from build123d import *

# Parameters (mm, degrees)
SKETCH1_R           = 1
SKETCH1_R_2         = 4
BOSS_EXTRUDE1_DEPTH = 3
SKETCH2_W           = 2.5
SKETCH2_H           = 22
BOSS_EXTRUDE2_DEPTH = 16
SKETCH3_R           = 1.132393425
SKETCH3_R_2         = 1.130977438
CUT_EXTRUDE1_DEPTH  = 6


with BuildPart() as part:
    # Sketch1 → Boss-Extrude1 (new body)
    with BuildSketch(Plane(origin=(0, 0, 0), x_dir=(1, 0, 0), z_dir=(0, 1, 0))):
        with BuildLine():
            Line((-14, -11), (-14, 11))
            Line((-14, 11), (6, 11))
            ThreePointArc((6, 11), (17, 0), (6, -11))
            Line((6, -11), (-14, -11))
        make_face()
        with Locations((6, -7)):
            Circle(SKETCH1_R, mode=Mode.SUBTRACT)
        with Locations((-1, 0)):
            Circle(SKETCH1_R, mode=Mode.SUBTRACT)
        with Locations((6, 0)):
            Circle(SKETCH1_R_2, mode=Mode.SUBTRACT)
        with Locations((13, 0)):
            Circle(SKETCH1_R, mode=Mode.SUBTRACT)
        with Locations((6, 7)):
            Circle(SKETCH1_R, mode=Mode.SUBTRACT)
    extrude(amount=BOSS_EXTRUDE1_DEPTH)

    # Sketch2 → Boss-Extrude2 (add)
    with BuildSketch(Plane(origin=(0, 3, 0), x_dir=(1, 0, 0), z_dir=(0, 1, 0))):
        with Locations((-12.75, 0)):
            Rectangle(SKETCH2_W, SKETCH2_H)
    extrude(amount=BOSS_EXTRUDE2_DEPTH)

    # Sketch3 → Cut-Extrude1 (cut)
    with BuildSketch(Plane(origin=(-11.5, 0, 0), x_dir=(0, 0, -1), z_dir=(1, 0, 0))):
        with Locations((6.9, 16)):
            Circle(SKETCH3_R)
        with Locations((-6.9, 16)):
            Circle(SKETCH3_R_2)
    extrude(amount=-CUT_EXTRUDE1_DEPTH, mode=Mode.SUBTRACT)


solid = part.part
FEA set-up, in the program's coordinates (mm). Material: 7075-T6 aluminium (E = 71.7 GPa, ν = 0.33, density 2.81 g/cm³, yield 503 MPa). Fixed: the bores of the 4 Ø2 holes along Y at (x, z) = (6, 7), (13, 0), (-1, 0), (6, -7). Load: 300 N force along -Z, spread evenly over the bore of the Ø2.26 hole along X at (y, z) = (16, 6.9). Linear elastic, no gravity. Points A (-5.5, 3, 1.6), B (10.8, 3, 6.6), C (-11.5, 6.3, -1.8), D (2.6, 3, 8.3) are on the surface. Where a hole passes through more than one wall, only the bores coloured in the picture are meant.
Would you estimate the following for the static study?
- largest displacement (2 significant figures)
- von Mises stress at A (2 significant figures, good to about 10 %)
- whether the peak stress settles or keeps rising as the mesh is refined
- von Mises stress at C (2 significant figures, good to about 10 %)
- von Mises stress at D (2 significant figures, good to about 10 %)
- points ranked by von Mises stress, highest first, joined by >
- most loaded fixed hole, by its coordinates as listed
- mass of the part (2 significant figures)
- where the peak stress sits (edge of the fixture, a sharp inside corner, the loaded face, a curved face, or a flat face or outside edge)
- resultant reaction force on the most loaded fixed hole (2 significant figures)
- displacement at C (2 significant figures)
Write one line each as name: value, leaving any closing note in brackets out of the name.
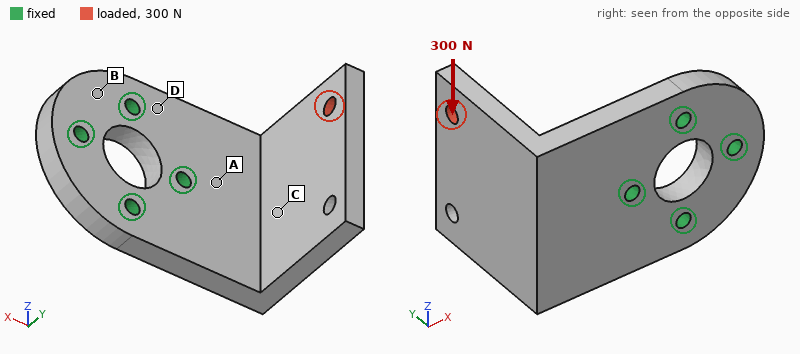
largest displacement: 0.20 mm
von Mises stress at A: 110 MPa
whether the peak stress settles or keeps rising as the mesh is refined: keeps rising
von Mises stress at C: 41 MPa
von Mises stress at D: 68 MPa
points ranked by von Mises stress, highest first, joined by >: A > D > C > B
most loaded fixed hole, by its coordinates as listed: (-1, 0)
mass of the part: 7.2 g
where the peak stress sits: edge of the fixture
resultant reaction force on the most loaded fixed hole: 330 N
displacement at C: 0.053 mm
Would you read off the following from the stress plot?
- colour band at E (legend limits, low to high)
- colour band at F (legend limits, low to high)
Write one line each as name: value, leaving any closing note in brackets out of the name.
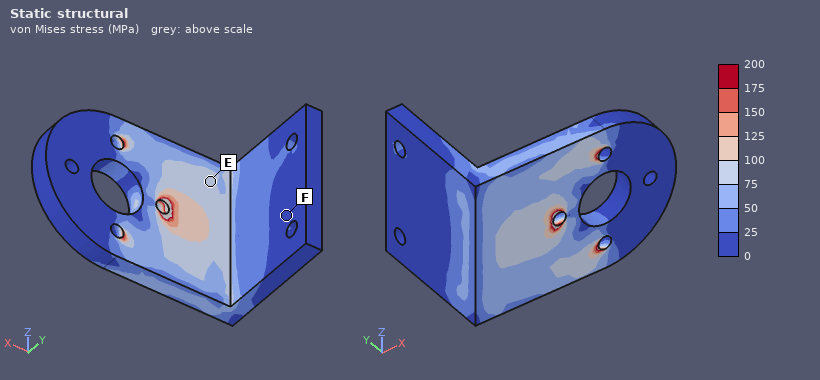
colour band at E: 75 to 100 MPa
colour band at F: 0 to 25 MPa
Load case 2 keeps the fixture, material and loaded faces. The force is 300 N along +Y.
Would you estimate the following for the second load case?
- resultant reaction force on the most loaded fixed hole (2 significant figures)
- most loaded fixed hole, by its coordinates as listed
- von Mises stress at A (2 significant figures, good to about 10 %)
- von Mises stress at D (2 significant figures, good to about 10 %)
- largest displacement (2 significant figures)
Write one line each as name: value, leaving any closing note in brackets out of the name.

resultant reaction force on the most loaded fixed hole: 470 N
most loaded fixed hole, by its coordinates as listed: (-1, 0)
von Mises stress at A: 85 MPa
von Mises stress at D: 69 MPa
largest displacement: 0.20 mm
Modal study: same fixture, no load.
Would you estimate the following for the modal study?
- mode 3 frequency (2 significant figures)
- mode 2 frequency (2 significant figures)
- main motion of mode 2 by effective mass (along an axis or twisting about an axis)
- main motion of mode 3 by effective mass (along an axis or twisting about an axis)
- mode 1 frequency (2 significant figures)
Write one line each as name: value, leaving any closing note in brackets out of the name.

mode 3 frequency: 9300 Hz
mode 2 frequency: 5300 Hz
main motion of mode 2 by effective mass: along Z
main motion of mode 3 by effective mass: along Y
mode 1 frequency: 3800 Hz
